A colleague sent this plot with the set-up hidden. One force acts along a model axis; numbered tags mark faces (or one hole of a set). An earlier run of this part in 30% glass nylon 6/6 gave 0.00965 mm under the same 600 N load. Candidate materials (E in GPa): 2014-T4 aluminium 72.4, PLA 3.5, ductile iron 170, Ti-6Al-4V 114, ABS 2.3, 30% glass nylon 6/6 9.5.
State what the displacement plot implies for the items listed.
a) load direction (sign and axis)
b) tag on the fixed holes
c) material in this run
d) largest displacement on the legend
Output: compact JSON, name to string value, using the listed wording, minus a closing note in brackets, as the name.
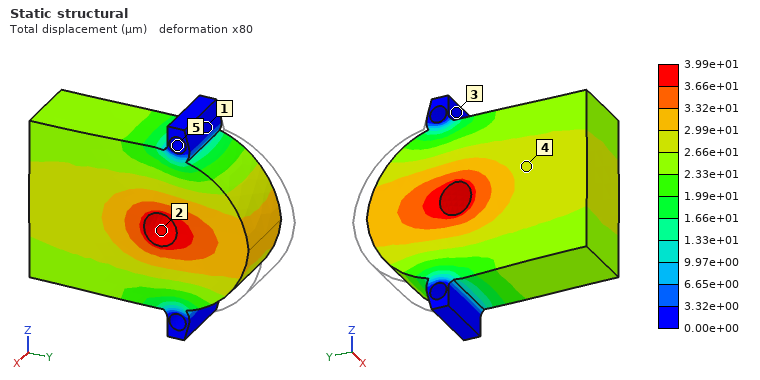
{"load direction": "-Y", "tag on the fixed holes": "5", "material in this run": "ABS", "largest displacement on the legend": "3.99e+01 µm"}
